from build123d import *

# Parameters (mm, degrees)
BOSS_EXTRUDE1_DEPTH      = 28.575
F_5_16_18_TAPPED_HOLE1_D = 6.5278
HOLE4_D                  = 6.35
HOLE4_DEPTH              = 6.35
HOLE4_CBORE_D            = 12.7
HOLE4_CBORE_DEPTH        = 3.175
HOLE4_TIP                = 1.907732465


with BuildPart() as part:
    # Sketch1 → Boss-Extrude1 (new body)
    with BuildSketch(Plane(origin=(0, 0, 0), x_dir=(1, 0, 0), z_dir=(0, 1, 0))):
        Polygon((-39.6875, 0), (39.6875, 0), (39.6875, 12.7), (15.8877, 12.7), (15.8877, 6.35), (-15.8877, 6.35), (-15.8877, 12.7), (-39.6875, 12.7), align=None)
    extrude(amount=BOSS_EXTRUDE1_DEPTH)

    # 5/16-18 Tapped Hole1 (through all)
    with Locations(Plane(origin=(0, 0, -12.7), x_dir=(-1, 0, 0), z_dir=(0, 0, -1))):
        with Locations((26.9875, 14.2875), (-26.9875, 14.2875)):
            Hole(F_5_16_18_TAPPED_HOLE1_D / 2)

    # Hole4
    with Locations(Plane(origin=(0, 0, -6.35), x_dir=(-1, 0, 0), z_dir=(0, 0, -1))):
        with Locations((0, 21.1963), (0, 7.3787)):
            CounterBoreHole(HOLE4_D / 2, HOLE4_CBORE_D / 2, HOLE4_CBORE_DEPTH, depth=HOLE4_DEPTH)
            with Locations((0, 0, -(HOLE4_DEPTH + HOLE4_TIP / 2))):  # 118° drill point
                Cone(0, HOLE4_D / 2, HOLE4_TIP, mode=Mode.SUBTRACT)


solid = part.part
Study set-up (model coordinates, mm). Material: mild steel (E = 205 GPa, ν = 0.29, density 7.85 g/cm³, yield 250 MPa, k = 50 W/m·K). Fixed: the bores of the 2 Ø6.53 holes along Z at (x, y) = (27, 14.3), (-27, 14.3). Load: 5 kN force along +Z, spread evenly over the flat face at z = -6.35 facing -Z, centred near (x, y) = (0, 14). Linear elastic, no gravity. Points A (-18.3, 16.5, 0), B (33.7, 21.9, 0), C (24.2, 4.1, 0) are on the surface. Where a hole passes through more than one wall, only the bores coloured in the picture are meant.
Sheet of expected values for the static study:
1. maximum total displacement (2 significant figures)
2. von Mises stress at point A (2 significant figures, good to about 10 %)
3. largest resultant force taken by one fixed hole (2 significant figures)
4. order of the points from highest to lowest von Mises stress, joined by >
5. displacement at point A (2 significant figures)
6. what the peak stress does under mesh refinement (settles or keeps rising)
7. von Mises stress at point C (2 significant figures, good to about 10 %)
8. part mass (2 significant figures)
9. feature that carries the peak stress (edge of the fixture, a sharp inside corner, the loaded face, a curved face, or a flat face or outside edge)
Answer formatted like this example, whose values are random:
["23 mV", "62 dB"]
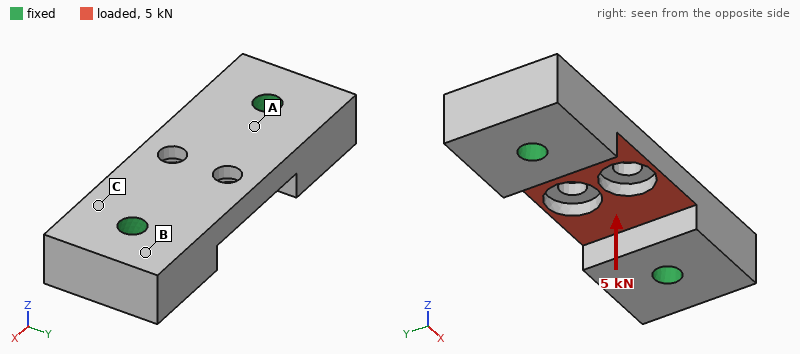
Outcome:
["13 µm", "37 MPa", "2.8 kN", "A > C > B", "2.6 µm", "keeps rising", "19 MPa", "170 g", "edge of the fixture"]
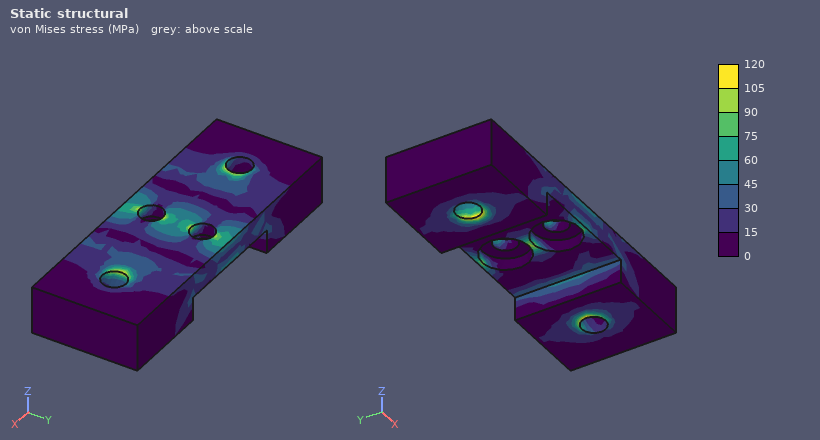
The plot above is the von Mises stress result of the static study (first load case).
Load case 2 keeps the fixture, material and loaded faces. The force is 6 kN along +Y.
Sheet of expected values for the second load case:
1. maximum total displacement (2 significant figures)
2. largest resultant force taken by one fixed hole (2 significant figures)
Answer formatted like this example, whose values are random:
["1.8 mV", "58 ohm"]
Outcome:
["8.6 µm", "3.0 kN"]
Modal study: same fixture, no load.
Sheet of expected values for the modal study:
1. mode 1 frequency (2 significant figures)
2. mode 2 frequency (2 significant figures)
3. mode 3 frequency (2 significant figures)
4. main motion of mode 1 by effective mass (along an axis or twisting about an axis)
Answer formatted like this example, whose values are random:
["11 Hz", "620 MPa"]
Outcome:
["18 kHz", "19 kHz", "23 kHz", "along Z"]
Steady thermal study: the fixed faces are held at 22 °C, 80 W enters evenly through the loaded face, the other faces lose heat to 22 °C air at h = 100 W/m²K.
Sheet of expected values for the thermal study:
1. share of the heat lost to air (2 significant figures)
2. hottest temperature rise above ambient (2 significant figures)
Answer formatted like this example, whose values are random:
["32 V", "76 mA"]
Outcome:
["16 %", "57 K"]
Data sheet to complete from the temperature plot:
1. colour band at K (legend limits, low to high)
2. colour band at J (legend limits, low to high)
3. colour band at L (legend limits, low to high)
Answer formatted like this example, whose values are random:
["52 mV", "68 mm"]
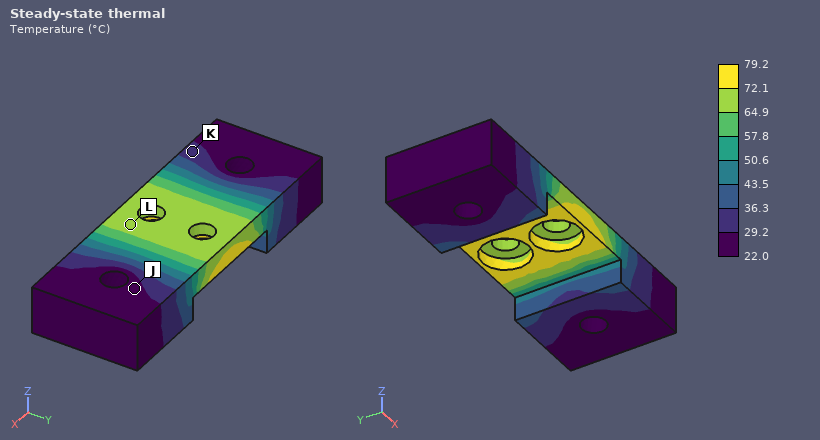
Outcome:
["29.2 to 36.3 °C", "22.0 to 29.2 °C", "64.9 to 72.1 °C"]
